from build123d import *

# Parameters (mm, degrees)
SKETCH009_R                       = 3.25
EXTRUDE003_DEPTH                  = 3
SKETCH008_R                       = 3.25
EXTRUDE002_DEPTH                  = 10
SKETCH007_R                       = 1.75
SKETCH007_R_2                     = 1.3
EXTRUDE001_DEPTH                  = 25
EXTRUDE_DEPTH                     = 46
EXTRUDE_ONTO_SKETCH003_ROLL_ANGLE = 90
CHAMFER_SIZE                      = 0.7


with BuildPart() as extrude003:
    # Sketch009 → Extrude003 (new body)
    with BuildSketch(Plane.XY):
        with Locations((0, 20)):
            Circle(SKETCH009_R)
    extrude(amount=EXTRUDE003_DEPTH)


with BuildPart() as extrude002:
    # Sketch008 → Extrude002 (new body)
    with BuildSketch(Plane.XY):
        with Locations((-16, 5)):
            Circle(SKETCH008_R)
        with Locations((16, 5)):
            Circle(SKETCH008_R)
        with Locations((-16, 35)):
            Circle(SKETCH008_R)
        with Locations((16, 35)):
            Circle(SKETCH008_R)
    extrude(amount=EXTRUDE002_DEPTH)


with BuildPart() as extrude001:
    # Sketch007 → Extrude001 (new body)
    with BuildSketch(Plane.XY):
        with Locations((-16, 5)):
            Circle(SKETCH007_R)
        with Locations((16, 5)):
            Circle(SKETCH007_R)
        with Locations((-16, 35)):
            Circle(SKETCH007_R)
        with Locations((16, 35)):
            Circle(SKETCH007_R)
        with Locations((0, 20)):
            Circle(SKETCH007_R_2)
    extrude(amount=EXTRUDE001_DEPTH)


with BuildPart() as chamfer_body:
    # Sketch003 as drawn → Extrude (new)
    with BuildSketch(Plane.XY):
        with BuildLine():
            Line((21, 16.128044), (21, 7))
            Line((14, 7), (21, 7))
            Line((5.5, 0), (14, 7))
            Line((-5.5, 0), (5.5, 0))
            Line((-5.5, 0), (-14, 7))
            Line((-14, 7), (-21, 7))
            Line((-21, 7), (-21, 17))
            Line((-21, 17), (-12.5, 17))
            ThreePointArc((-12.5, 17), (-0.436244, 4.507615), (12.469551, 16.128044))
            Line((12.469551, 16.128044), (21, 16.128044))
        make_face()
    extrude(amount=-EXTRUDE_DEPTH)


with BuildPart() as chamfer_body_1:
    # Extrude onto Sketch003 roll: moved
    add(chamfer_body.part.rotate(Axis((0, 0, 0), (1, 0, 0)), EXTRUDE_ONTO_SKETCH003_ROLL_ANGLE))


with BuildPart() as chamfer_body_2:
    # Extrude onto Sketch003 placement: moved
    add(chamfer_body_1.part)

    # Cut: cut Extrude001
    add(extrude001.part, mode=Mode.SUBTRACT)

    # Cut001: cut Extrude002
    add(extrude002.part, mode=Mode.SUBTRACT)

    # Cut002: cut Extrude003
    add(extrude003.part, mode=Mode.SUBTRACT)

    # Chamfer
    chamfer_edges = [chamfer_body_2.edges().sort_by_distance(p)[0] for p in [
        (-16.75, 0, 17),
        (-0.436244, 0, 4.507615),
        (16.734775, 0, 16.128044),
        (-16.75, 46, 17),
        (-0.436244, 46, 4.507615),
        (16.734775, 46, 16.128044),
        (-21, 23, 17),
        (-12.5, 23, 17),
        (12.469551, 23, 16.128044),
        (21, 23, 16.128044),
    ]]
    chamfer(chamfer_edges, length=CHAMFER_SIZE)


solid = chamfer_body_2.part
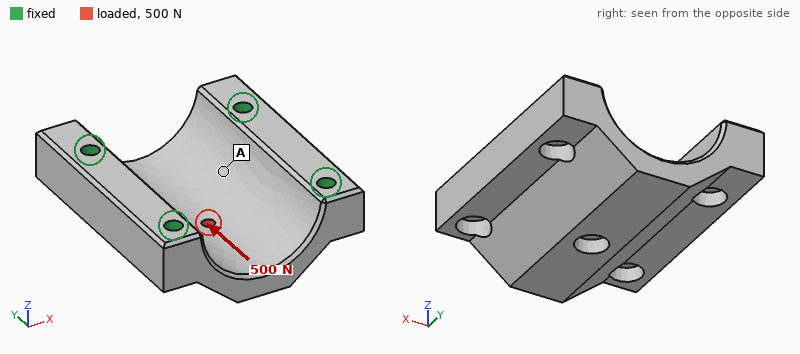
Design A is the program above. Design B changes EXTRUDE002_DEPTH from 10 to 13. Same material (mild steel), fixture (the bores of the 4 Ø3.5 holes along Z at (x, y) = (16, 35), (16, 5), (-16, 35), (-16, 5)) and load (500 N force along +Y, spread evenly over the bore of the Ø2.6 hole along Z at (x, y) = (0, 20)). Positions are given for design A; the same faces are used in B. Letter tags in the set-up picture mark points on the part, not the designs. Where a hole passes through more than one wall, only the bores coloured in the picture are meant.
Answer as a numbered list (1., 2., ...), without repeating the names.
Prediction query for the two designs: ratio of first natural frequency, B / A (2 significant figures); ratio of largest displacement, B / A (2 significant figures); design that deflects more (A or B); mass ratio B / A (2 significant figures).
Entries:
1. 0.68
2. 1.1
3. B
4. 0.98
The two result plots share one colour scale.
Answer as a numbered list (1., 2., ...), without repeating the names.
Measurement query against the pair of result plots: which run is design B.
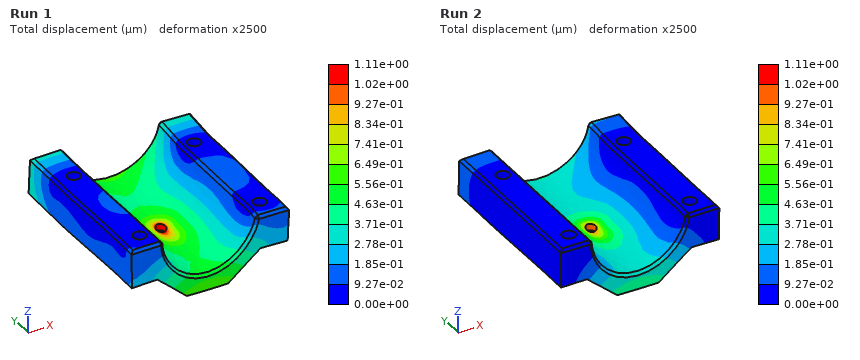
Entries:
1. Run 1
